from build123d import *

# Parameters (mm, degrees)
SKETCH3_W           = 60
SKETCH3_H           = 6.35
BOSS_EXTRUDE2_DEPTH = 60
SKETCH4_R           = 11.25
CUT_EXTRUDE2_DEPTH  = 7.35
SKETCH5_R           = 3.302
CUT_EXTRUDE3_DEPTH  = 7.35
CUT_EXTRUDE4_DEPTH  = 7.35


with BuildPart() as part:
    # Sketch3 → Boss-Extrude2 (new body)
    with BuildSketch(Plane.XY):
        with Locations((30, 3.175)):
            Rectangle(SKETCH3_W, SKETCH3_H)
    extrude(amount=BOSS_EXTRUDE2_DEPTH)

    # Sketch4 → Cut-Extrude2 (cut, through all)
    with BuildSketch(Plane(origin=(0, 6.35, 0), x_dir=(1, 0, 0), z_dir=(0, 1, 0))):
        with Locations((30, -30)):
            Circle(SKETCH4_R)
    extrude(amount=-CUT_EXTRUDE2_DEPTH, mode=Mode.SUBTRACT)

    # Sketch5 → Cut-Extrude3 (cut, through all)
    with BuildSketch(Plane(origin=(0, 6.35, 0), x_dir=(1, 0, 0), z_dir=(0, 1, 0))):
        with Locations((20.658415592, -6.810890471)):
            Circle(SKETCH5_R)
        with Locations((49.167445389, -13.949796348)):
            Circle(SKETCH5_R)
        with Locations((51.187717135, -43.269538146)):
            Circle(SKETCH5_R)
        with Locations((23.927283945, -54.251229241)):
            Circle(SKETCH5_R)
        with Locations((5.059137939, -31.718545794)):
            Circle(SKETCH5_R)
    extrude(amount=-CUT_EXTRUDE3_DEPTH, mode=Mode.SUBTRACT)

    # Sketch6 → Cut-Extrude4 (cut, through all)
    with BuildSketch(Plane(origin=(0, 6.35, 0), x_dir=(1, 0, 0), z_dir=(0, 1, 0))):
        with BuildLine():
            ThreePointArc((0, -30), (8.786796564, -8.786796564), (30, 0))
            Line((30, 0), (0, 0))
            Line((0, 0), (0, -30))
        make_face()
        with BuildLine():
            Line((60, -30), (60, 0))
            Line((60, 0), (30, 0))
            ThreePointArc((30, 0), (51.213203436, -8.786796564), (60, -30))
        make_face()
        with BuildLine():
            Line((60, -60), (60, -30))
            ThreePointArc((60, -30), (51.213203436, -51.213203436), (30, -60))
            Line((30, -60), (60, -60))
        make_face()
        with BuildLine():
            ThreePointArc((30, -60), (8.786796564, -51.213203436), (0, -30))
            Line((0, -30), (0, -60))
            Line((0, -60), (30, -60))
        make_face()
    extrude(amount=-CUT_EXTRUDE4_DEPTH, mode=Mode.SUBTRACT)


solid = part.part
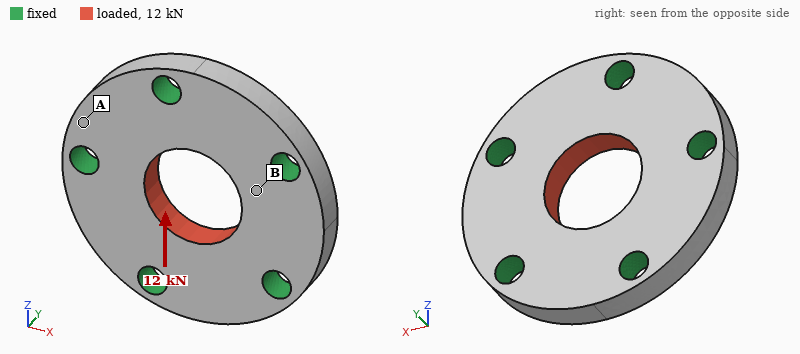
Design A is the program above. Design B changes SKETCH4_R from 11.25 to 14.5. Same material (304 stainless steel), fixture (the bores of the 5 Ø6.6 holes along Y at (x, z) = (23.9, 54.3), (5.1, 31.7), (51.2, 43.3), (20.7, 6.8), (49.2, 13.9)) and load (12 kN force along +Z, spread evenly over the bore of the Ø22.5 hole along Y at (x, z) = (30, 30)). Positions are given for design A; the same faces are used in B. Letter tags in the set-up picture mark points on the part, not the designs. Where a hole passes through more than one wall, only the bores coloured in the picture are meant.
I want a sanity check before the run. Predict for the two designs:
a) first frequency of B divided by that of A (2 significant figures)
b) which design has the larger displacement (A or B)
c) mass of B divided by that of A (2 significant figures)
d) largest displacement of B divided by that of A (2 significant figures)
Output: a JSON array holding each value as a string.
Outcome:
["1.1", "A", "0.88", "0.91"]
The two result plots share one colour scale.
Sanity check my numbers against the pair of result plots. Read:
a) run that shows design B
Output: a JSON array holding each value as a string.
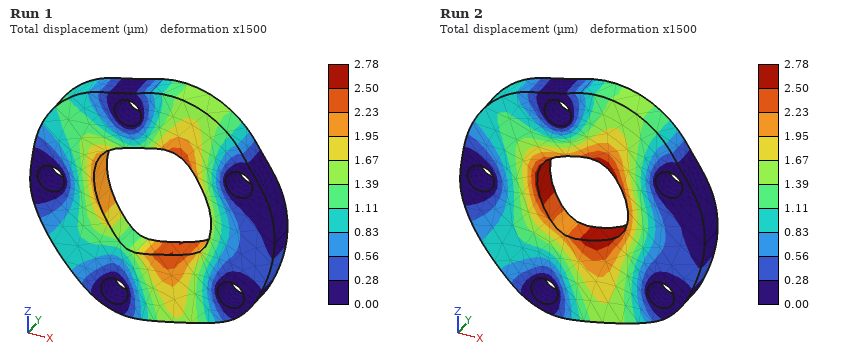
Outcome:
["Run 1"]
